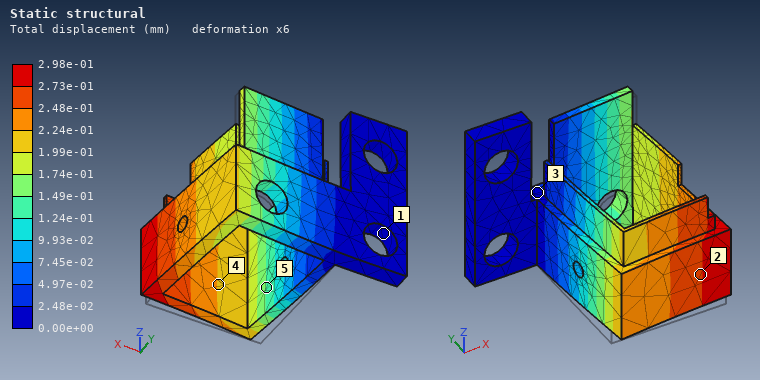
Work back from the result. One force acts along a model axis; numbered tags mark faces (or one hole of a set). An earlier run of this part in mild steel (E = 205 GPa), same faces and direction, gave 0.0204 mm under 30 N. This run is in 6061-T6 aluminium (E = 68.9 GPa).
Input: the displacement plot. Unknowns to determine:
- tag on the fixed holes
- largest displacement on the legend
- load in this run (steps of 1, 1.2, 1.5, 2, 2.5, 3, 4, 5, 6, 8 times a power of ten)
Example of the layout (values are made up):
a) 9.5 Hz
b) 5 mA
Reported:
a) 1
b) 2.98e-01 mm
c) 150 N
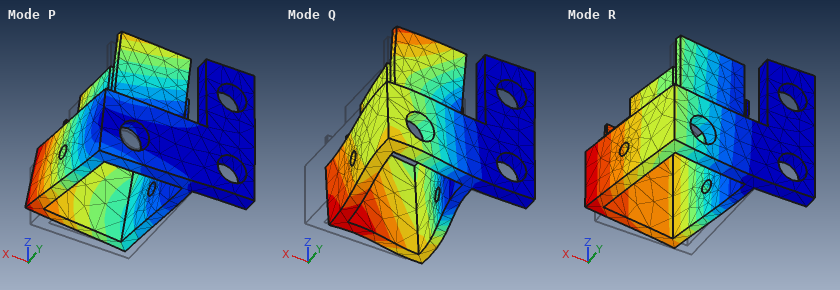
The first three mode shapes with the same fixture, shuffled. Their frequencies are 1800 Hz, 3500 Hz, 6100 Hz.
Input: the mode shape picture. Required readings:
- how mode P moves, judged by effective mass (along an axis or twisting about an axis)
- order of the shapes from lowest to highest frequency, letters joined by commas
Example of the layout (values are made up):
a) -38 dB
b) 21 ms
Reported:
a) along Z
b) R, P, Q
